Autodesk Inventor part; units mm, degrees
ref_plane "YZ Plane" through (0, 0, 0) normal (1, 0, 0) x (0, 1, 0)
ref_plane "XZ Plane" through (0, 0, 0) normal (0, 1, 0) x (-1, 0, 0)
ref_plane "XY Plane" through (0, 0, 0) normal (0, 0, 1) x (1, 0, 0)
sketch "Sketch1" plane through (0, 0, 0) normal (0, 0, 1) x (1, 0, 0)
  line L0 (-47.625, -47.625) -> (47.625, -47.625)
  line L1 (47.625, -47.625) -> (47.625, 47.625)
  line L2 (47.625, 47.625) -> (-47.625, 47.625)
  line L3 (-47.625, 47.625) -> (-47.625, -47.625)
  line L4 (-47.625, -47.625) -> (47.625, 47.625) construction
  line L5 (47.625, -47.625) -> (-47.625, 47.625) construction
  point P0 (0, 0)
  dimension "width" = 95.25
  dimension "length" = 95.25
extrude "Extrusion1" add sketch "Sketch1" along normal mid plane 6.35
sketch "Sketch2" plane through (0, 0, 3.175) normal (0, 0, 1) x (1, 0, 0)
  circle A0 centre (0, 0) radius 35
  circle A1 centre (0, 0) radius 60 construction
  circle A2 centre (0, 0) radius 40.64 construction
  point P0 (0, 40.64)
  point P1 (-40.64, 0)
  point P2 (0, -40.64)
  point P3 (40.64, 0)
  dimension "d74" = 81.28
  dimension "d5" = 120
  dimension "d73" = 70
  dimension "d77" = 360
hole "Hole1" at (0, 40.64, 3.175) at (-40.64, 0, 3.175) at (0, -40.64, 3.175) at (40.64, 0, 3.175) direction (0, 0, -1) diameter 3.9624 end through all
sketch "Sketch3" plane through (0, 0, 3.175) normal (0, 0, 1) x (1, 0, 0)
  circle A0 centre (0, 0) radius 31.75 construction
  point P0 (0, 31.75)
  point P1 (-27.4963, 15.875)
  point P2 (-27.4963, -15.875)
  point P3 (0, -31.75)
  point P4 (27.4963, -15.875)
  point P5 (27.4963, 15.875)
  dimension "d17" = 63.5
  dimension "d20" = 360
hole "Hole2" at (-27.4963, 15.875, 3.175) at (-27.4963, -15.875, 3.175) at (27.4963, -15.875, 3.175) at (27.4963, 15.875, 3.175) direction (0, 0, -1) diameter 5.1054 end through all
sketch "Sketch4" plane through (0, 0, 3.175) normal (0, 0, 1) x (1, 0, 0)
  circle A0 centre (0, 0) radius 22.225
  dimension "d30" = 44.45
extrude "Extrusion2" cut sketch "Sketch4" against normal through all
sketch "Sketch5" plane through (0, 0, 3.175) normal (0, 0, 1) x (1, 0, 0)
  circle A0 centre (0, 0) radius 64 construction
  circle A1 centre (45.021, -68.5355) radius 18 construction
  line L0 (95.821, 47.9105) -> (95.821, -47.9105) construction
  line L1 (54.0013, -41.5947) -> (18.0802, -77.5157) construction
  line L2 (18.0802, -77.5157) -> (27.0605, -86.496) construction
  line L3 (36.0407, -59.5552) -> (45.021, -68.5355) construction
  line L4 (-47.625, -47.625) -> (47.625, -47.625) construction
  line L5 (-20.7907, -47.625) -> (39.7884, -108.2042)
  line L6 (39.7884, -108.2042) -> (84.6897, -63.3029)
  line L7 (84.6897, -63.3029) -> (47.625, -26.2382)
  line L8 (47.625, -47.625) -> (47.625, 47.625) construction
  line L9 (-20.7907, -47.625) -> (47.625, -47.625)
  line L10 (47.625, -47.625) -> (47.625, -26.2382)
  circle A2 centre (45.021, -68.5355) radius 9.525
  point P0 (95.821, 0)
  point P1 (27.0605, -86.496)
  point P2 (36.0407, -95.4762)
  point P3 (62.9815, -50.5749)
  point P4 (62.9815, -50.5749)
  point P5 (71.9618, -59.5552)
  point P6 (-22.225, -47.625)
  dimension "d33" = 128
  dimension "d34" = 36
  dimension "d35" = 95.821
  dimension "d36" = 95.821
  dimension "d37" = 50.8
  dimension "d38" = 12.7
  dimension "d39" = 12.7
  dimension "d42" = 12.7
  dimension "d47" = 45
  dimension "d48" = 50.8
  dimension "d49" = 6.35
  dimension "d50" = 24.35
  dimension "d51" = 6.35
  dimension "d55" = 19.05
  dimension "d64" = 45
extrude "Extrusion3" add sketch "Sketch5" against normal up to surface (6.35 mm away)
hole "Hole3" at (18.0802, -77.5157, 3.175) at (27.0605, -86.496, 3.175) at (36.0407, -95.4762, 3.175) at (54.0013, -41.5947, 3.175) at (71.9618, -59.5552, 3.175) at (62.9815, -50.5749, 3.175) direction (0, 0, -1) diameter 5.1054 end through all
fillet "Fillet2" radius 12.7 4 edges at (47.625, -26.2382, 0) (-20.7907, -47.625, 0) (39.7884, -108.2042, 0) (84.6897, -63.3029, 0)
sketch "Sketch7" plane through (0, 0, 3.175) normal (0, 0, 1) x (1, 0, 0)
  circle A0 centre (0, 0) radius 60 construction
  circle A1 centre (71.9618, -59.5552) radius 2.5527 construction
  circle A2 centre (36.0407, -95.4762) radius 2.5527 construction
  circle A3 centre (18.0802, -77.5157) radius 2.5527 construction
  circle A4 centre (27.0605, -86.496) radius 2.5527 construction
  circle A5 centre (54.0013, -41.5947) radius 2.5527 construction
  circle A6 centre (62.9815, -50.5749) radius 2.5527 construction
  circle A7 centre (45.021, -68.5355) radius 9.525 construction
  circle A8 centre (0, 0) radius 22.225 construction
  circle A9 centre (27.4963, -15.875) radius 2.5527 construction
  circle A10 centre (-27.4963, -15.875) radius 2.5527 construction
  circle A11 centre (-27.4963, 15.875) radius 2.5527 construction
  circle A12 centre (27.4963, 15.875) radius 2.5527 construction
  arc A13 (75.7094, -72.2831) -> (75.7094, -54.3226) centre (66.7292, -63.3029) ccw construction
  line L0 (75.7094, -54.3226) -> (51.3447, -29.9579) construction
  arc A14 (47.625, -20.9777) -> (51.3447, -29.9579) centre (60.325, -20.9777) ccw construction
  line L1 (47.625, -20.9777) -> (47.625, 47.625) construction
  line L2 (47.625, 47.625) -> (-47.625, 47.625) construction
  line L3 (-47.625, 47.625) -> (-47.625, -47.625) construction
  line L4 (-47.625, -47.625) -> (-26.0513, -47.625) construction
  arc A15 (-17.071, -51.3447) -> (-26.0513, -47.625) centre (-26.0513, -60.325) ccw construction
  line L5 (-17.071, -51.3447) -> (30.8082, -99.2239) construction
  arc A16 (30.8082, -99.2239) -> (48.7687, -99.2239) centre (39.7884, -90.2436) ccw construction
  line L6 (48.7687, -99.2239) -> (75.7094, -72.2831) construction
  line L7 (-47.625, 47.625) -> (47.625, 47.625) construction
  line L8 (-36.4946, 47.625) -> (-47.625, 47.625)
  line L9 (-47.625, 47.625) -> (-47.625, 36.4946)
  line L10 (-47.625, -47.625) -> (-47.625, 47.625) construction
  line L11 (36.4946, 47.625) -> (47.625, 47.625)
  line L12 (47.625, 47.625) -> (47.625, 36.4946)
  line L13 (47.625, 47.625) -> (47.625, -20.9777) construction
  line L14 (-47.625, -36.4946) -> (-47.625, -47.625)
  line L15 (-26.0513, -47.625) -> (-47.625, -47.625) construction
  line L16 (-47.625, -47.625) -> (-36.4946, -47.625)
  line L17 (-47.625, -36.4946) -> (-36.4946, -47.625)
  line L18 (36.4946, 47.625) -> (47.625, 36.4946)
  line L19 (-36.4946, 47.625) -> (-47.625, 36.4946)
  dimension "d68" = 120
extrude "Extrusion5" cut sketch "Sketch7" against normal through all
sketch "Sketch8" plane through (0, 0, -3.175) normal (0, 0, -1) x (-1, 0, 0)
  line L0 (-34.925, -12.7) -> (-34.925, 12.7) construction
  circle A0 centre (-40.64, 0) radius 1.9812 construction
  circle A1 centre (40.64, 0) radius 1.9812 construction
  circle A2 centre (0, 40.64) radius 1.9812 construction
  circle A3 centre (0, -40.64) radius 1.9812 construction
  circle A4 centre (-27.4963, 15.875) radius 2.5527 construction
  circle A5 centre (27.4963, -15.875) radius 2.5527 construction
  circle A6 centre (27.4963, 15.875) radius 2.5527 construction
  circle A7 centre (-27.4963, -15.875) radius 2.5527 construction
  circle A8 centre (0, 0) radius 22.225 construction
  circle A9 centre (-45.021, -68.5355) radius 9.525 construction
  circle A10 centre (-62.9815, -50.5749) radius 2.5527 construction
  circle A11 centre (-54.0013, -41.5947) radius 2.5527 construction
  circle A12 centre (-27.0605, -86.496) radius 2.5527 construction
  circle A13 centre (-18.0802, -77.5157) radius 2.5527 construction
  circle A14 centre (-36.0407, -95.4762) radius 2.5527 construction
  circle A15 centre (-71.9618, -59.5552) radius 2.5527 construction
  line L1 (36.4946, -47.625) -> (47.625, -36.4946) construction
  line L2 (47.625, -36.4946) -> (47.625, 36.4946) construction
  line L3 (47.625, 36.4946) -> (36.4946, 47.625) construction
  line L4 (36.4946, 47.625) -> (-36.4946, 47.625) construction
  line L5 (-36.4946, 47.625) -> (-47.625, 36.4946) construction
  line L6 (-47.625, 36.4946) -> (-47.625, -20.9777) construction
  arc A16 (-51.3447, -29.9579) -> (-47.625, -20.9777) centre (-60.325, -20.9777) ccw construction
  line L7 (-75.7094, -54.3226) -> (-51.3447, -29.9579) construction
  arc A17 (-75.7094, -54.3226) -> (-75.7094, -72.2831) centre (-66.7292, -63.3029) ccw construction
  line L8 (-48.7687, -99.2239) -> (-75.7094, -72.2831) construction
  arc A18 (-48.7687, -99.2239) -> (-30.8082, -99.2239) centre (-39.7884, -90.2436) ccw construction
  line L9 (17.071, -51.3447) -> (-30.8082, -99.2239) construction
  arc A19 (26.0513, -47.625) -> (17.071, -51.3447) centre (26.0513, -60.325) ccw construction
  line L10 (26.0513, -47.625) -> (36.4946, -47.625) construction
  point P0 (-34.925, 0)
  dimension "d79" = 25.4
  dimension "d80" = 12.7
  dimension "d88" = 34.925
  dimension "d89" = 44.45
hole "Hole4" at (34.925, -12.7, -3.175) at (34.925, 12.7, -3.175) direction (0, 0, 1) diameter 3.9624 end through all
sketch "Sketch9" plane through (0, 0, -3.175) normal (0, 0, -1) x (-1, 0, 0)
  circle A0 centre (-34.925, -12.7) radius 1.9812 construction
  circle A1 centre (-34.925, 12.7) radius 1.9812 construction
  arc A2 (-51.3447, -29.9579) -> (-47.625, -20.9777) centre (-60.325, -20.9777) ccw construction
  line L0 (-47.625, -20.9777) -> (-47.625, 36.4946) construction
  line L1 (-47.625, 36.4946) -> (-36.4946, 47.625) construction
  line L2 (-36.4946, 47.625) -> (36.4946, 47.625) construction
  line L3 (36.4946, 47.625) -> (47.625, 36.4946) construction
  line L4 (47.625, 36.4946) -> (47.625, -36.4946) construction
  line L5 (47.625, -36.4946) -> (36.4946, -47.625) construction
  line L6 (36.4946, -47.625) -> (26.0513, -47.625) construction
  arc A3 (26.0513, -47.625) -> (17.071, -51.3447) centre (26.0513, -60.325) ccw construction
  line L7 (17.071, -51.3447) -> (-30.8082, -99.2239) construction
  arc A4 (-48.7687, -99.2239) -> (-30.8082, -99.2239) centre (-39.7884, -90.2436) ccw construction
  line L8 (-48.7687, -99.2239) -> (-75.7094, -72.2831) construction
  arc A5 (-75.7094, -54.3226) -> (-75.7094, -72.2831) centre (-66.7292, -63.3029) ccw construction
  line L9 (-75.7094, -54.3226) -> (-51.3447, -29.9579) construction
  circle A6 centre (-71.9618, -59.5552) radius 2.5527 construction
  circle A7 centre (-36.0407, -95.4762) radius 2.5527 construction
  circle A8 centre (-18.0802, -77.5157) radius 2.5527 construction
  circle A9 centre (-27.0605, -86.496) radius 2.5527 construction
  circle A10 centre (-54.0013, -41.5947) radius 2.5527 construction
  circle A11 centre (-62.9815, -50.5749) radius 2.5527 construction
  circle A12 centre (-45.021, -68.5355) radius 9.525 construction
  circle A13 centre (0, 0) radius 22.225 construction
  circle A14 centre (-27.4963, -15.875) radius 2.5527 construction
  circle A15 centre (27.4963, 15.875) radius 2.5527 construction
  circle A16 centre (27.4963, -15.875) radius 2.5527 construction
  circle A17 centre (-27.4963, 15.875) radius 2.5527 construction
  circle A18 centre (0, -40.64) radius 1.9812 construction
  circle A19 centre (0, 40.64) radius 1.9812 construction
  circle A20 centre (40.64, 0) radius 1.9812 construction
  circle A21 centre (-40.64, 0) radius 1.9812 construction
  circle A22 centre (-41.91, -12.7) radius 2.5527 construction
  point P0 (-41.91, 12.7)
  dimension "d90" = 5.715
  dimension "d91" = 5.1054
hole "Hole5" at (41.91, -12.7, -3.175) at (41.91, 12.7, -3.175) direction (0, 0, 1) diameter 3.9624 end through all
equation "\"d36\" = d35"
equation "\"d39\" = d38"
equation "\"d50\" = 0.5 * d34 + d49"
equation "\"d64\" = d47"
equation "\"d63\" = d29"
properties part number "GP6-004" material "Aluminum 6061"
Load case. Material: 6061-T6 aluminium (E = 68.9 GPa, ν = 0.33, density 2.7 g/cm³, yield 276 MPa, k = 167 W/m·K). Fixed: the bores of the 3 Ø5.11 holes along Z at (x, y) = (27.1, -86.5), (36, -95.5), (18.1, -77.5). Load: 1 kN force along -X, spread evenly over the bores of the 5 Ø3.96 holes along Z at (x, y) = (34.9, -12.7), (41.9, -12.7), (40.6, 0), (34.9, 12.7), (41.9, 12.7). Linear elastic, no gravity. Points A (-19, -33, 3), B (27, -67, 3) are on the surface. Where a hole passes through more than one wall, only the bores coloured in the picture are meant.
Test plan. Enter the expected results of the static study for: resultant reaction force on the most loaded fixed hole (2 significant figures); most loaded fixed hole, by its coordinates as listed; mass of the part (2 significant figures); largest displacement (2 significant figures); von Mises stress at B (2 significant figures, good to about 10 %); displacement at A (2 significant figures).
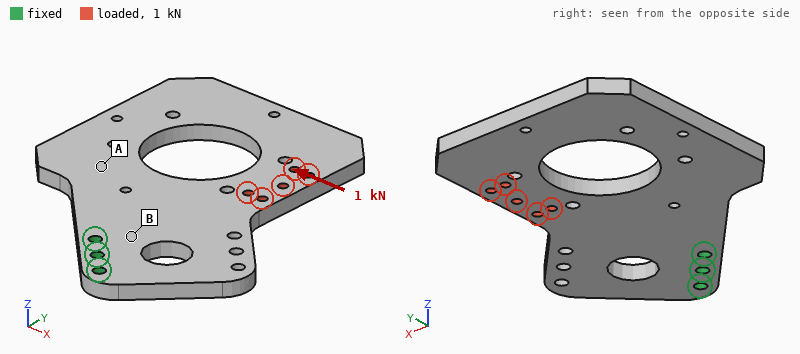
3.2 kN
(18.1, -77.5)
180 g
0.17 mm
24 MPa
0.072 mm
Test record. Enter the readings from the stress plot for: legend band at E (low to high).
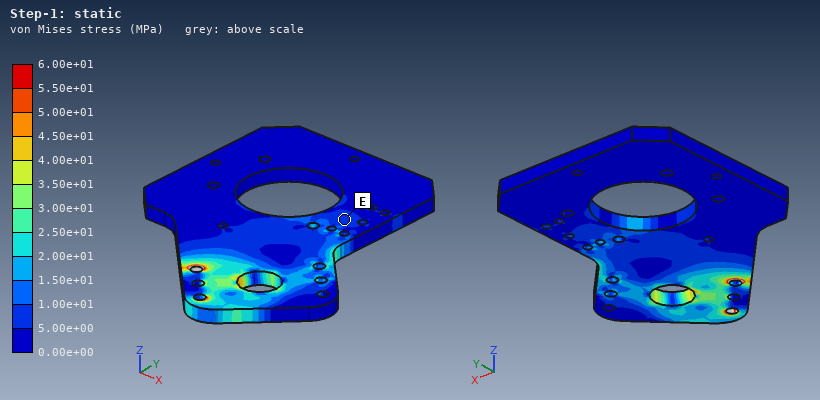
5.00e+00 to 1.00e+01 MPa
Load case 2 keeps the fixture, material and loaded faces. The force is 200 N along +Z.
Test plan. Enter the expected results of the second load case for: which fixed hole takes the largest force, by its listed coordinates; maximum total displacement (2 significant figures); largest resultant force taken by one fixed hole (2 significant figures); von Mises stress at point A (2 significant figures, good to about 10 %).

(18.1, -77.5)
0.87 mm
370 N
7.1 MPa
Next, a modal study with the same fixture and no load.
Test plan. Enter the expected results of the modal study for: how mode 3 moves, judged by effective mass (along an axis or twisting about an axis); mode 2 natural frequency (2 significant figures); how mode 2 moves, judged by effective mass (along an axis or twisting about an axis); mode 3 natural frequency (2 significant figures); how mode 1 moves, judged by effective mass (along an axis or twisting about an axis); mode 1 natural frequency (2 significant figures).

along X
620 Hz
twisting about Y
1200 Hz
along Z
250 Hz
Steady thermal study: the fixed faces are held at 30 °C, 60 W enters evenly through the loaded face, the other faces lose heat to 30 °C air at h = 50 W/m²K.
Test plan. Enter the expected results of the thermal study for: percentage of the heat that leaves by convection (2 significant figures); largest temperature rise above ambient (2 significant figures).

55 %
62 K
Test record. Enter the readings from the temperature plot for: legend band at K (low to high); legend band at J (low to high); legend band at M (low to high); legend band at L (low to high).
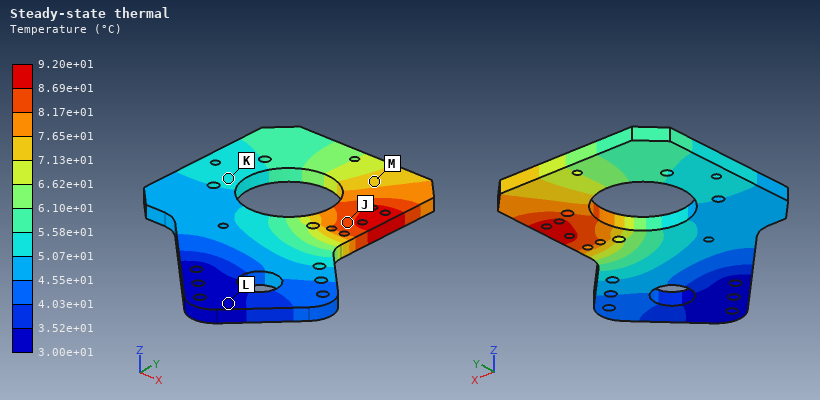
5.07e+01 to 5.58e+01 °C
8.17e+01 to 8.69e+01 °C
7.13e+01 to 7.65e+01 °C
3.00e+01 to 3.52e+01 °C
